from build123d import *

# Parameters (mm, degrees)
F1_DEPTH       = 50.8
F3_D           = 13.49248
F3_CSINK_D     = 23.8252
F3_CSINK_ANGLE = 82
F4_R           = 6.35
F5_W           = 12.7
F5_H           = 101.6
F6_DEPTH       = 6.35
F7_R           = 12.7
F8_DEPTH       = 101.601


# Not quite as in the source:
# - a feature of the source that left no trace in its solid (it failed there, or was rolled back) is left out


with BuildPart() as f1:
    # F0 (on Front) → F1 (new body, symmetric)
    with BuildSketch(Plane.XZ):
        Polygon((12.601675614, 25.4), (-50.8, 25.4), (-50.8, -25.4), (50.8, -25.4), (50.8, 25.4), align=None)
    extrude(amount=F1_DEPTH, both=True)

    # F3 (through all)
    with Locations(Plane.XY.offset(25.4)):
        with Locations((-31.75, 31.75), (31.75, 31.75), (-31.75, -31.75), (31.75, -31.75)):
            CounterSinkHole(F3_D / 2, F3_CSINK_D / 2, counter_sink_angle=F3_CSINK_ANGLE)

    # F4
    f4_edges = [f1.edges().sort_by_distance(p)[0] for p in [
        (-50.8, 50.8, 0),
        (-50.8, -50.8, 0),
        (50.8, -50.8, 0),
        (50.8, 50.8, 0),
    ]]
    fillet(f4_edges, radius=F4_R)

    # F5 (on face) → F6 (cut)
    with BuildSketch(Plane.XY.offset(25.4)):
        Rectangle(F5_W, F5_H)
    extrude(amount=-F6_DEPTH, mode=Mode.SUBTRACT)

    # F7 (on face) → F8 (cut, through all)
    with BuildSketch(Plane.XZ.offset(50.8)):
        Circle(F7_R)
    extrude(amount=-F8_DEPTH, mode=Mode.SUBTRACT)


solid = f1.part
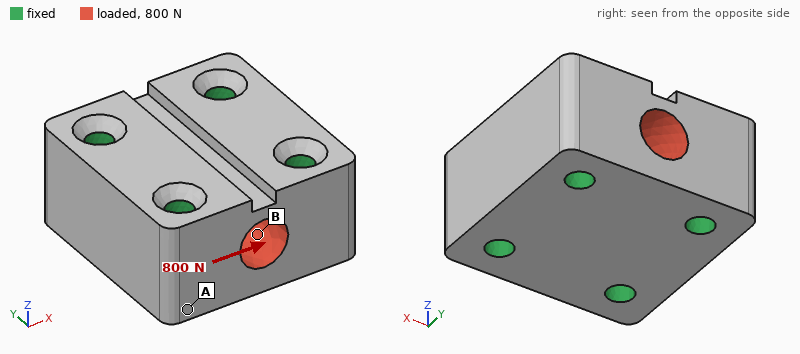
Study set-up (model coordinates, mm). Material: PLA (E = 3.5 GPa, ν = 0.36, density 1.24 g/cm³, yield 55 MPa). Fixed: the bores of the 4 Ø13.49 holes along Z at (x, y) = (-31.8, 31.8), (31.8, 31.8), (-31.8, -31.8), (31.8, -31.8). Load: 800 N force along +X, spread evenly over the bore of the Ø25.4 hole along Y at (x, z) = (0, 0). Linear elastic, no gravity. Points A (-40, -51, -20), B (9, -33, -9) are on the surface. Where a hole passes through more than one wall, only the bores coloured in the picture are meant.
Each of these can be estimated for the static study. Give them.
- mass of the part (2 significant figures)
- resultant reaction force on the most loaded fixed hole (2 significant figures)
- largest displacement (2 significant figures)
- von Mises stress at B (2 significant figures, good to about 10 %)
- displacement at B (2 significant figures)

530 g
200 N
1.3 µm
0.16 MPa
0.64 µm
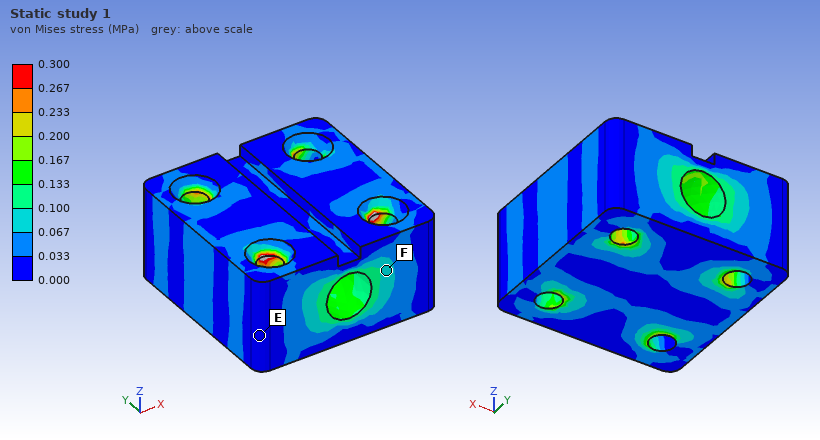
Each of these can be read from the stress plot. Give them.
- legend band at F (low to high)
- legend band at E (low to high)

0.067 to 0.100 MPa
0.000 to 0.033 MPa
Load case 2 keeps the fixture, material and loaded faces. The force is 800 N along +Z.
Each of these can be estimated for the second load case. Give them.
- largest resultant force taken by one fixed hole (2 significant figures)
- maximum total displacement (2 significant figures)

200 N
3.7 µm
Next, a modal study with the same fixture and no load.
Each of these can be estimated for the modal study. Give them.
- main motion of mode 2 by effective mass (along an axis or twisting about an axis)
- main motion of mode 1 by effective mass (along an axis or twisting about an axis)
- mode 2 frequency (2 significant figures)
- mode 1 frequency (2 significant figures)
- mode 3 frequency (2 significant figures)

along X
along Z
7200 Hz
6600 Hz
7600 Hz
